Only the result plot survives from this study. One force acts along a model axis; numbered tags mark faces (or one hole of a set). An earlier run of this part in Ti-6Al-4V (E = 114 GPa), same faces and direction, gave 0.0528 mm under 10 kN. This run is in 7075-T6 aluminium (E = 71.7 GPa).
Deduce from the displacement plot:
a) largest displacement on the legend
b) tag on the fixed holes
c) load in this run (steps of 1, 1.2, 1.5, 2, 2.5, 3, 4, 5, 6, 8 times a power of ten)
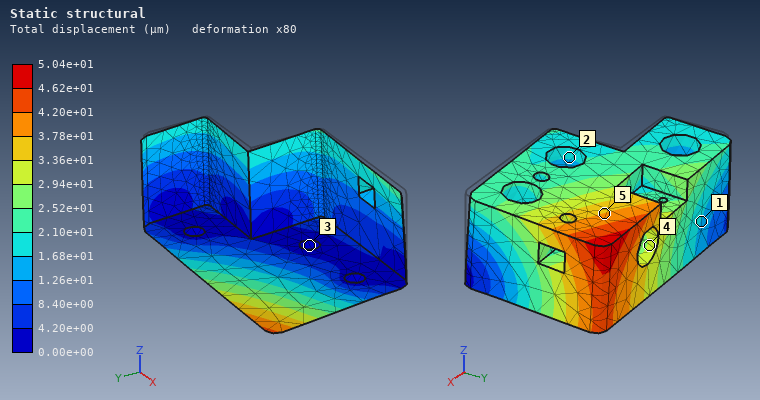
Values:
5.04e+01 µm
3
6 kN
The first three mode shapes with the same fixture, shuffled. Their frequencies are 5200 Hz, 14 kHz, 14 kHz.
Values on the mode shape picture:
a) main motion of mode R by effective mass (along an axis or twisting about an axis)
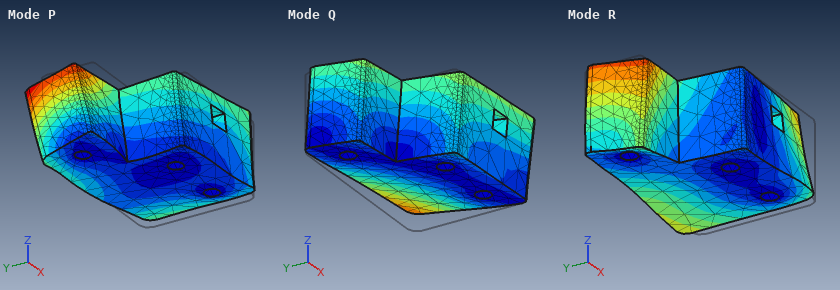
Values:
along X
